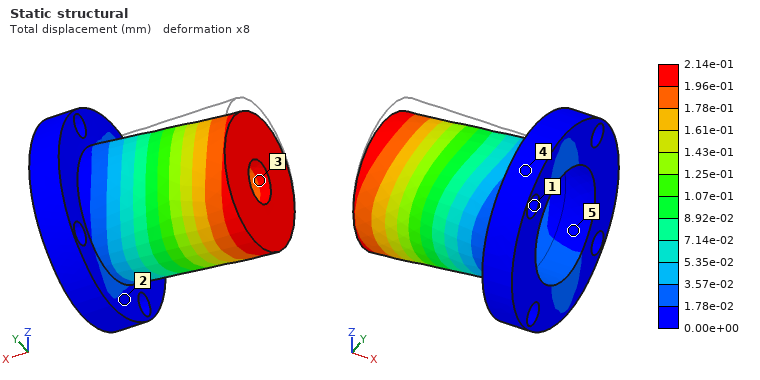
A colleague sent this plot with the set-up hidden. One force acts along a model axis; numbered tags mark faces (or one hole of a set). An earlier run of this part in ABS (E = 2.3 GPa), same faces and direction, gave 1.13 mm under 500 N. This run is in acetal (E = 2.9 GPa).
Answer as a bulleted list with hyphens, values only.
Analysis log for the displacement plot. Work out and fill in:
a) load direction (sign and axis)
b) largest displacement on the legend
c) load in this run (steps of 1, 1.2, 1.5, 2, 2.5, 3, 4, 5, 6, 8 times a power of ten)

- -Z
- 2.14e-01 mm
- 120 N
